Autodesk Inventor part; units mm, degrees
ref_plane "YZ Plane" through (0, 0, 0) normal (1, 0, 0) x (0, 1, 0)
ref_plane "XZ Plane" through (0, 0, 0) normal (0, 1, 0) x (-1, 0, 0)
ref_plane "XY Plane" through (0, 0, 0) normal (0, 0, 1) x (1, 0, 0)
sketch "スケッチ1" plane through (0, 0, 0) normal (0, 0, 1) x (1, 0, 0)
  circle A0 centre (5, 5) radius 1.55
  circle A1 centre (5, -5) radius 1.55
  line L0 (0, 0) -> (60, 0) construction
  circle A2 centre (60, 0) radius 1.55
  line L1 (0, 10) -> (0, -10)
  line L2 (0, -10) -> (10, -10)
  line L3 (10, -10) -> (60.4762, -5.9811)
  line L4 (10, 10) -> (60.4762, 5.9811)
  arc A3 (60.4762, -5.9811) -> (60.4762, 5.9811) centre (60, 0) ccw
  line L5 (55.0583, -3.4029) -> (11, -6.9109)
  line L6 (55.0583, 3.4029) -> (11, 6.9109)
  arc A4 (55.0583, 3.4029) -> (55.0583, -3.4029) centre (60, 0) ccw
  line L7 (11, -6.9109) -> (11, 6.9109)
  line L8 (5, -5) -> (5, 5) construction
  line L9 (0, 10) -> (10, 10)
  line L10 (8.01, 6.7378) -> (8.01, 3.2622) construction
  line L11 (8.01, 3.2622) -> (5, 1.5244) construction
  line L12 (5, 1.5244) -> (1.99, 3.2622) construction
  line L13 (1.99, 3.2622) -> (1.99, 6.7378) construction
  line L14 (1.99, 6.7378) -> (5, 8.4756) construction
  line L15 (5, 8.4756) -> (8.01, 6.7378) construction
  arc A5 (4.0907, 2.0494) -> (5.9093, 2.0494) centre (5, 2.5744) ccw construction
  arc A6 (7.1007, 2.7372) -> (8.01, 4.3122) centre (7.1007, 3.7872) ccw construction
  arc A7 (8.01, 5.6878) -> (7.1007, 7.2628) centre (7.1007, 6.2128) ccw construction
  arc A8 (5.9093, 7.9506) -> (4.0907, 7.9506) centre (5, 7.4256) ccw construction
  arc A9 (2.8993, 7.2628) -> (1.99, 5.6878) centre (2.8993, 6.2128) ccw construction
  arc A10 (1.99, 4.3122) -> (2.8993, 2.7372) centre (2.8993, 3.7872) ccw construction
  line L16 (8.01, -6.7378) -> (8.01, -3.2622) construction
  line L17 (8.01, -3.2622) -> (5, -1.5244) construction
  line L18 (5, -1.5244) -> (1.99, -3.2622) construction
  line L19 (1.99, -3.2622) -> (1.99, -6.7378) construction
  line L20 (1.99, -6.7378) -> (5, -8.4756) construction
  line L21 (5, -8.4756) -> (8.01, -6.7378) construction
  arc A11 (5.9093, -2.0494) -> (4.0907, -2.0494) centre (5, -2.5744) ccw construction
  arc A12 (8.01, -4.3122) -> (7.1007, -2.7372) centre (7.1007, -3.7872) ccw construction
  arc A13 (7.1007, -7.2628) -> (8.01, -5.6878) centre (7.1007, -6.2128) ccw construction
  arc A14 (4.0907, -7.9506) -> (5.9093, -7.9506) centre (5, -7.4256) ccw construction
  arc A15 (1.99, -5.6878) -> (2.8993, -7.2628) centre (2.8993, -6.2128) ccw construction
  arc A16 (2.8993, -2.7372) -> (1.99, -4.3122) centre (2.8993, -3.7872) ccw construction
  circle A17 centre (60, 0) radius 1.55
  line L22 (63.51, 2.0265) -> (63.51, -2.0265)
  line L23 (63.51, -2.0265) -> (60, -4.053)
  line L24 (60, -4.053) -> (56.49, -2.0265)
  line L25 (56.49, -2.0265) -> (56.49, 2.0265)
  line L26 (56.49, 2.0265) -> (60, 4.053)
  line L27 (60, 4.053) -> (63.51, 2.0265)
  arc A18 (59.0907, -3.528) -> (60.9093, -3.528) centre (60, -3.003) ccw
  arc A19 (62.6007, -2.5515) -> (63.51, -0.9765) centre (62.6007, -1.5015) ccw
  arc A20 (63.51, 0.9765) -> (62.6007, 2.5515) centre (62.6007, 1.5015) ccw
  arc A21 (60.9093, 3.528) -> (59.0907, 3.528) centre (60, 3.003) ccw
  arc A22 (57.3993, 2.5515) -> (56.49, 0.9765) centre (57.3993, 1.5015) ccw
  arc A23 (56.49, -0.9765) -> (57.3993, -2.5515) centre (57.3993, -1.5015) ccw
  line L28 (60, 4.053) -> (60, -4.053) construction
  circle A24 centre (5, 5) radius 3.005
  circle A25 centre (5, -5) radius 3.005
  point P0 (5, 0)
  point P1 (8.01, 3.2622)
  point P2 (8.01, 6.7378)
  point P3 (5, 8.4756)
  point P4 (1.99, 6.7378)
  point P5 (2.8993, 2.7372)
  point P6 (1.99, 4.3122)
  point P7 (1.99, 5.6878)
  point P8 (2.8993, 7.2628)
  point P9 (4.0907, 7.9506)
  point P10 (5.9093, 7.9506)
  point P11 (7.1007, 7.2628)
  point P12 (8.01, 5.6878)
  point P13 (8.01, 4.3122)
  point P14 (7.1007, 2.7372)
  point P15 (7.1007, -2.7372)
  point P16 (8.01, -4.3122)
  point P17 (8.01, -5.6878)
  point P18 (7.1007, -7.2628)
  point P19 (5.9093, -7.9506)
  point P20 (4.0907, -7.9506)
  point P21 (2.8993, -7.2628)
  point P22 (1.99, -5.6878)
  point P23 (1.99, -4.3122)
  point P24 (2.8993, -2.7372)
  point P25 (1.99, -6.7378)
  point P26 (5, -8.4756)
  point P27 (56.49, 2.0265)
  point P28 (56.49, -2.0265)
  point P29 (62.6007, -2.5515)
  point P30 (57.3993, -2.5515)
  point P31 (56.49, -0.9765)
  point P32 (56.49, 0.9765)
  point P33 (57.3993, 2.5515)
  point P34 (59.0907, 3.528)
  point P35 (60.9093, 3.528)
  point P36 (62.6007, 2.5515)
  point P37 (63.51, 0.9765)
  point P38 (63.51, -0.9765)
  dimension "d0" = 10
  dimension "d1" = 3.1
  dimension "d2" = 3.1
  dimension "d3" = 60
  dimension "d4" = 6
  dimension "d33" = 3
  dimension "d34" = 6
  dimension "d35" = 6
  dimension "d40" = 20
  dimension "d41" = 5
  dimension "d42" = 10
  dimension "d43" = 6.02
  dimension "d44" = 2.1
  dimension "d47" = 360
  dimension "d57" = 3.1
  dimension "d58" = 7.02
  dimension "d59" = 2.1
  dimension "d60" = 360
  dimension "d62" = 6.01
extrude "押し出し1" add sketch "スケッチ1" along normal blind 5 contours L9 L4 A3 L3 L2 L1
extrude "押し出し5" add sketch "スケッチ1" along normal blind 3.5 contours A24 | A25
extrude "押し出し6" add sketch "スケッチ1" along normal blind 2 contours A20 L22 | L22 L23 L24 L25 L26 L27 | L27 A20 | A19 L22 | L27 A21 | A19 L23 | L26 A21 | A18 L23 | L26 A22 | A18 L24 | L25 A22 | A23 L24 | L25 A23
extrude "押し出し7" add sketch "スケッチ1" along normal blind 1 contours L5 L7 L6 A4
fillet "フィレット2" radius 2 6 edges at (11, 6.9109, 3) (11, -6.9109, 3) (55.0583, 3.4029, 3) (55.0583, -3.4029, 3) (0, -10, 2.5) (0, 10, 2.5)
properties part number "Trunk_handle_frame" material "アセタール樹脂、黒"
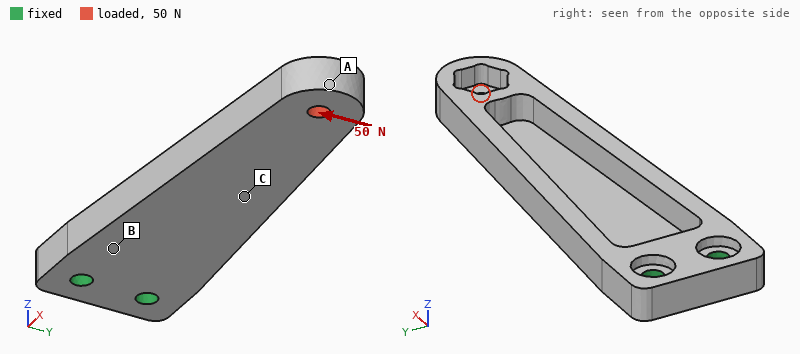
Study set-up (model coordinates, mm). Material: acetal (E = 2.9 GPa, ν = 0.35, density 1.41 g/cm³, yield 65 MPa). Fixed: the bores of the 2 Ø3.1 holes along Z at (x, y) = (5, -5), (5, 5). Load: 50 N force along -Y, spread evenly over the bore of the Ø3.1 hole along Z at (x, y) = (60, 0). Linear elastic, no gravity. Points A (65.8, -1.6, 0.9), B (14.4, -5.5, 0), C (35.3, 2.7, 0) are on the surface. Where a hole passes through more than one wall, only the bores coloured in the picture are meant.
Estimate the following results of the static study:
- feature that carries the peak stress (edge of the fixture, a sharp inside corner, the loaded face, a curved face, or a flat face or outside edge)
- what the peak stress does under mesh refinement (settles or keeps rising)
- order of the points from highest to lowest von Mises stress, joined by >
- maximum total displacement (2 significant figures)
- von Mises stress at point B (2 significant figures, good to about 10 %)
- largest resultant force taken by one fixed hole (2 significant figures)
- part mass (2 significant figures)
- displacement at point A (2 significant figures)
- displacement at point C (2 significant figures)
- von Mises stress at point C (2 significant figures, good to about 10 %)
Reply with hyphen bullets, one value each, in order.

- edge of the fixture
- keeps rising
- B > C > A
- 0.82 mm
- 8.2 MPa
- 230 N
- 4.5 g
- 0.75 mm
- 0.25 mm
- 4.9 MPa
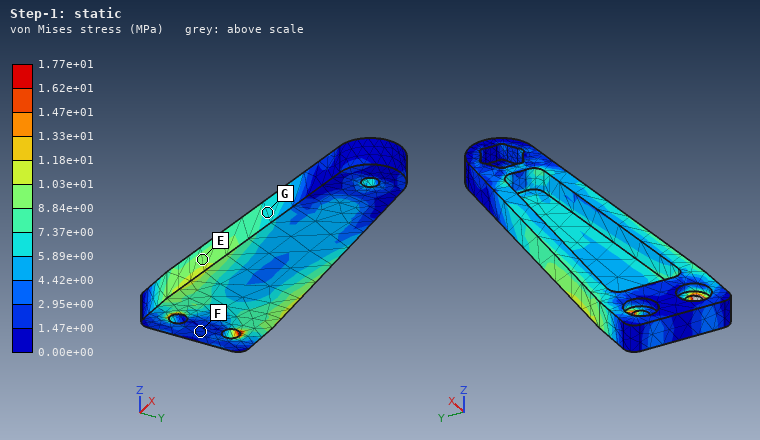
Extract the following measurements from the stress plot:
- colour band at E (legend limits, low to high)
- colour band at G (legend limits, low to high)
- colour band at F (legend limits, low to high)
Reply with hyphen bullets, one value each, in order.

- 8.84e+00 to 1.03e+01 MPa
- 5.89e+00 to 7.37e+00 MPa
- 1.47e+00 to 2.95e+00 MPa
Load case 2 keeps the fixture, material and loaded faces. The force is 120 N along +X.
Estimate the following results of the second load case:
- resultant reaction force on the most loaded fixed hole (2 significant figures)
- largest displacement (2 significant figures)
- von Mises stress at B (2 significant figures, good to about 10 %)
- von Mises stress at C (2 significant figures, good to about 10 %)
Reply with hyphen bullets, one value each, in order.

- 60 N
- 0.72 mm
- 4.9 MPa
- 5.5 MPa
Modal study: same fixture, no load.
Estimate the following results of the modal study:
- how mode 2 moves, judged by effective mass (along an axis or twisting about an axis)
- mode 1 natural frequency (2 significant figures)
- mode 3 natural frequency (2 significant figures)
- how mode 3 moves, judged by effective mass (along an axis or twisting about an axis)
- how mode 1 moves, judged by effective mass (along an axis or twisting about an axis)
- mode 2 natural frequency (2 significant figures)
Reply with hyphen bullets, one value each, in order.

- along Y
- 340 Hz
- 1600 Hz
- along Y
- along Z
- 1000 Hz
